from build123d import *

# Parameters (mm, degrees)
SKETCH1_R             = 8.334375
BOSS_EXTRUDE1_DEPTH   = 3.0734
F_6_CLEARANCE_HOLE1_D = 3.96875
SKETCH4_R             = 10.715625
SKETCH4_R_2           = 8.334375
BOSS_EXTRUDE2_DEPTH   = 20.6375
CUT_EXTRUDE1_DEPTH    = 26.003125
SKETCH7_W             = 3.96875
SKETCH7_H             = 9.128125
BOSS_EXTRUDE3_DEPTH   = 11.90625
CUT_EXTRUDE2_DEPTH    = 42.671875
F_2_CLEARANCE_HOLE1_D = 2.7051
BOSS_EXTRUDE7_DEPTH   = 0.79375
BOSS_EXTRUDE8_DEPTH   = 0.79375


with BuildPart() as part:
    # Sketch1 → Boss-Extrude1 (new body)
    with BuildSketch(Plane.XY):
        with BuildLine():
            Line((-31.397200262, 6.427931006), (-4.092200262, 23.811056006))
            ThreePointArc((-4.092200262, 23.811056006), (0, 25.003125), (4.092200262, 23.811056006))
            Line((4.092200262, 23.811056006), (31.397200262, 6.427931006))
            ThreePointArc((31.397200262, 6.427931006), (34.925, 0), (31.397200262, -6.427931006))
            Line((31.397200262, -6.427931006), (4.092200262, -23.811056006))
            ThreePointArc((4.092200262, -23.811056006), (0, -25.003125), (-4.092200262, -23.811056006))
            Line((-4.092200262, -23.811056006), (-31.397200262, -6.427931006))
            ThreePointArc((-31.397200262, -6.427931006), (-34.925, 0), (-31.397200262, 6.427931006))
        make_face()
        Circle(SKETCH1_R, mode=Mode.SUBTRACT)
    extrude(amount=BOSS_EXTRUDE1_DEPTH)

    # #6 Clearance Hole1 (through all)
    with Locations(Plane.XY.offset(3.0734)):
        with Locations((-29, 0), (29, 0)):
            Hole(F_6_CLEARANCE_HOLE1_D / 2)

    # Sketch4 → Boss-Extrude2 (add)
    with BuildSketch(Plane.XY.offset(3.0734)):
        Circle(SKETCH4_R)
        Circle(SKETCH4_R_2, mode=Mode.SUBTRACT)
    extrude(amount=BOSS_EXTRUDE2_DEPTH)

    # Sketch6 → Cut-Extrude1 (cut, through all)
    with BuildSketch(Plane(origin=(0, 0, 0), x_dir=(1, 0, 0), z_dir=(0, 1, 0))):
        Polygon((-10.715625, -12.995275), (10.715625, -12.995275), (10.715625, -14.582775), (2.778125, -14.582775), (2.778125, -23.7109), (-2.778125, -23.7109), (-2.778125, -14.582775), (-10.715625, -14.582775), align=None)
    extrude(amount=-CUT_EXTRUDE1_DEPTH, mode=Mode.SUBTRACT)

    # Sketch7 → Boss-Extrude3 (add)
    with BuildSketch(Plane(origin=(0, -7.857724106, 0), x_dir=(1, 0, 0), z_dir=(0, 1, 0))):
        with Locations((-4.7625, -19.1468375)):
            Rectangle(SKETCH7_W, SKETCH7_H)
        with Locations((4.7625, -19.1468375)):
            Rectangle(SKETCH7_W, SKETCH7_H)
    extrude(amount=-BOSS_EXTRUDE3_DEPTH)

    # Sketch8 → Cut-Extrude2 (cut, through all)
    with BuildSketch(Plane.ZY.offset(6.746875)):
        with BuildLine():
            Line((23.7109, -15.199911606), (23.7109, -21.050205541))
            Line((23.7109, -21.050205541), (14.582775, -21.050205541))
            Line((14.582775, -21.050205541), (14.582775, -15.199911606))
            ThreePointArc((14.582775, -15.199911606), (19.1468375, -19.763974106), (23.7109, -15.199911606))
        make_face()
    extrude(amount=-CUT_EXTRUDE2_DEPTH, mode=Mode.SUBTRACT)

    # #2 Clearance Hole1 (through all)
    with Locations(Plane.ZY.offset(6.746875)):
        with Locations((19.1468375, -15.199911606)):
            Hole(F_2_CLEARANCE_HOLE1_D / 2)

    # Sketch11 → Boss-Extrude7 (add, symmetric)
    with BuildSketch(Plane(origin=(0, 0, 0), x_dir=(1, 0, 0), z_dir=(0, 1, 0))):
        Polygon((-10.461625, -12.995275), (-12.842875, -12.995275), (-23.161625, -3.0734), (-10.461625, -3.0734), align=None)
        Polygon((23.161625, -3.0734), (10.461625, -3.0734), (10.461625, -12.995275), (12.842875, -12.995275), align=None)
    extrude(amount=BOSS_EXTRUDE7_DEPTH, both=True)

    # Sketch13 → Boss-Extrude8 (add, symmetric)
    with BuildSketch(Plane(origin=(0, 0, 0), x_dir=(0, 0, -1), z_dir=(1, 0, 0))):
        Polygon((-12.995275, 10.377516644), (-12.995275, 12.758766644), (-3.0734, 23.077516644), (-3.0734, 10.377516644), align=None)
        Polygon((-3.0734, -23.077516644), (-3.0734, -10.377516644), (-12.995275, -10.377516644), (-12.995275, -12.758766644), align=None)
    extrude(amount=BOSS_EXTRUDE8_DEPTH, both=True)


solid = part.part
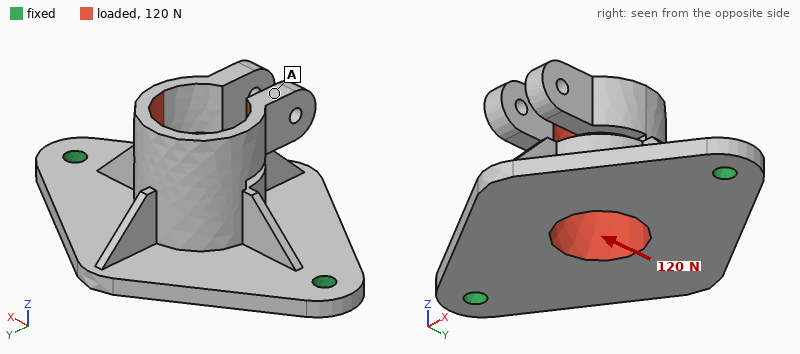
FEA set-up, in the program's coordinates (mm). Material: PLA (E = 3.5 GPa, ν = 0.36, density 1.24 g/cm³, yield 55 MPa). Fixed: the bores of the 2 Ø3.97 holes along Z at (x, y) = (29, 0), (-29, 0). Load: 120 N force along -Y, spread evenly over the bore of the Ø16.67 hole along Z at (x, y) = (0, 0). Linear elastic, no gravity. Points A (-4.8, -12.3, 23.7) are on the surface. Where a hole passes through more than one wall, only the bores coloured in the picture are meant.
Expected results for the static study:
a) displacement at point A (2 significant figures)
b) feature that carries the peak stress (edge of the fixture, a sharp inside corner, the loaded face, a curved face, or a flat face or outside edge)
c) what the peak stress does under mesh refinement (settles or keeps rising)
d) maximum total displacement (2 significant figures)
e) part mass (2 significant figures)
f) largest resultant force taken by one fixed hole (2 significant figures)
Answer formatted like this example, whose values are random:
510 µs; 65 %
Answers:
0.93 mm; edge of the fixture; keeps rising; 1.0 mm; 12 g; 61 N
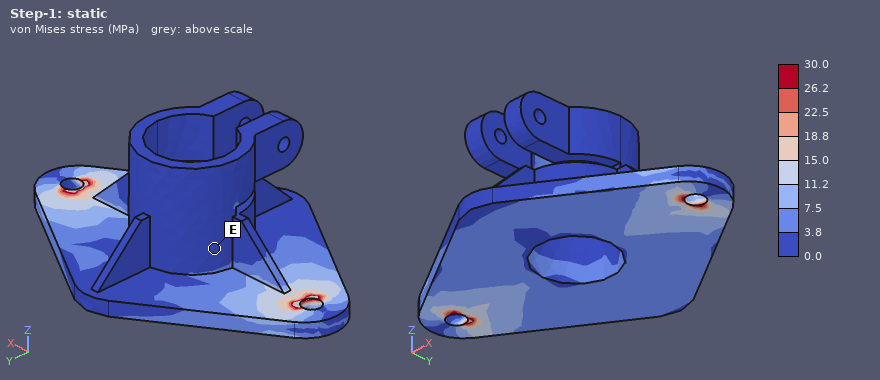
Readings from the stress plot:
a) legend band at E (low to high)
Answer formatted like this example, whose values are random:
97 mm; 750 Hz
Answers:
0.0 to 3.8 MPa
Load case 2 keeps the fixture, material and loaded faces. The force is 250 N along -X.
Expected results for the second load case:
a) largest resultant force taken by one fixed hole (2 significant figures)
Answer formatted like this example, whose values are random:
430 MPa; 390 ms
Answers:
140 N
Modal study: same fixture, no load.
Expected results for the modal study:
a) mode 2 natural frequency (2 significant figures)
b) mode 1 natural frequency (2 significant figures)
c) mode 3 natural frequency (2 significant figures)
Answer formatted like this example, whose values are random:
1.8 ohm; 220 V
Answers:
780 Hz; 640 Hz; 840 Hz
